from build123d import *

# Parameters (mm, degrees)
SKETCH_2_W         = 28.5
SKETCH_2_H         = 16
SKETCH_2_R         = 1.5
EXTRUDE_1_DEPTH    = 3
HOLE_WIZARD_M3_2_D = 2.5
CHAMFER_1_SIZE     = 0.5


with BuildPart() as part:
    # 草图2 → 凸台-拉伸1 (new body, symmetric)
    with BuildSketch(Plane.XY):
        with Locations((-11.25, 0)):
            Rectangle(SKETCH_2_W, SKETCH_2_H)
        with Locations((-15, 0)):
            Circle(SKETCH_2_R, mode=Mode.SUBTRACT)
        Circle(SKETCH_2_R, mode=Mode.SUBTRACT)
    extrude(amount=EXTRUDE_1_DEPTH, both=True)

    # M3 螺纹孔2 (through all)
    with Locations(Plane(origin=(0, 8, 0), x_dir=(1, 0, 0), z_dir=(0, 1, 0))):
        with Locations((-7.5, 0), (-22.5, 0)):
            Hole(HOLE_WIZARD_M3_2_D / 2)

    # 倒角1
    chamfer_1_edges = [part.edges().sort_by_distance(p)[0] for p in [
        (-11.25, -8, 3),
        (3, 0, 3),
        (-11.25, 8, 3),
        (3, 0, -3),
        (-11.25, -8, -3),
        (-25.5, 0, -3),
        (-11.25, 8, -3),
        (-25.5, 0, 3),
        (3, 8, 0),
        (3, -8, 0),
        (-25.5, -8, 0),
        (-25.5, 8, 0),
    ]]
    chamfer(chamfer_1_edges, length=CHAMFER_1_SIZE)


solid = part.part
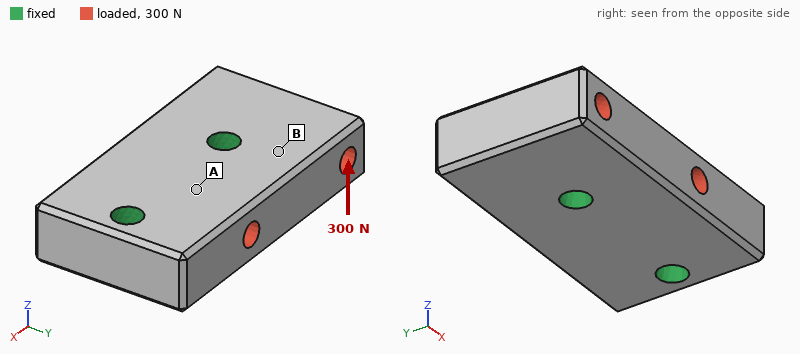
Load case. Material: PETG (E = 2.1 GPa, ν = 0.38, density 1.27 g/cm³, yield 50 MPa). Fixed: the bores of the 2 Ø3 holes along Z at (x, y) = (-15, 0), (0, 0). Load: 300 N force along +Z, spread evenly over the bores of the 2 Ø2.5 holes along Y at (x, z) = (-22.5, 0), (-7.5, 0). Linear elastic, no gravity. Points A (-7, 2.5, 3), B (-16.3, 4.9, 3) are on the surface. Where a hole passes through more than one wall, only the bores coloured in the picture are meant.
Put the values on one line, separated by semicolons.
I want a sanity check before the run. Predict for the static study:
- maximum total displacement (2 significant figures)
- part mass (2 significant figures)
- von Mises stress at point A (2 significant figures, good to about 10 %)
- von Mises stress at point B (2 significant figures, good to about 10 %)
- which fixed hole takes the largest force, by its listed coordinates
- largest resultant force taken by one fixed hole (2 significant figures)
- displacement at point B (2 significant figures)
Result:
92 µm; 3.1 g; 2.6 MPa; 5.7 MPa; (-15, 0); 240 N; 20 µm
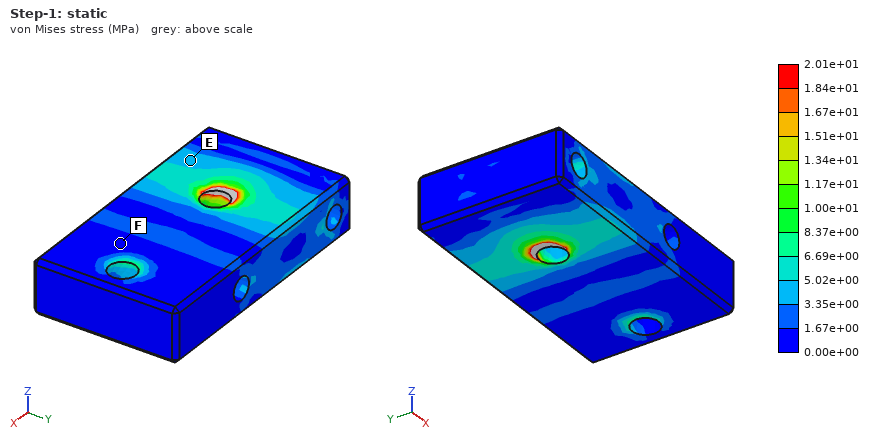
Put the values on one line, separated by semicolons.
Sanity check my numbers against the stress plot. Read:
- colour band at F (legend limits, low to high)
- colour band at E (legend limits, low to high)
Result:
0.00e+00 to 1.67e+00 MPa; 3.35e+00 to 5.02e+00 MPa
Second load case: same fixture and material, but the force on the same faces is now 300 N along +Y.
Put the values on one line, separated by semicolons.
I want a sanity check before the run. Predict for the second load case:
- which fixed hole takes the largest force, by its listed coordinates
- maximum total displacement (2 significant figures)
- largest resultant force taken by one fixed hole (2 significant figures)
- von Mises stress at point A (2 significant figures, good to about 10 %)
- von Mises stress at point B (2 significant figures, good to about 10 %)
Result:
(-15, 0); 53 µm; 280 N; 1.3 MPa; 2.6 MPa
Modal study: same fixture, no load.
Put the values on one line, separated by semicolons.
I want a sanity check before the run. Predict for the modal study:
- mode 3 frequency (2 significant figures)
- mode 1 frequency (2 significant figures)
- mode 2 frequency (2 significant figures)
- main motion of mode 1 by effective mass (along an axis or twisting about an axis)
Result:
10 kHz; 8700 Hz; 10 kHz; along Z
